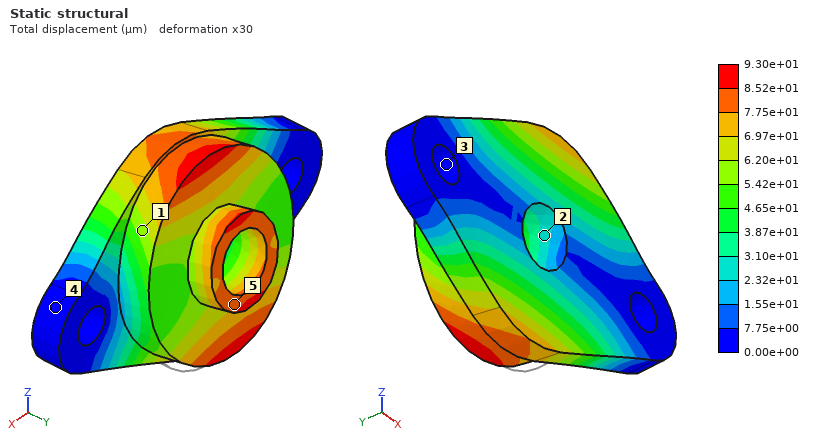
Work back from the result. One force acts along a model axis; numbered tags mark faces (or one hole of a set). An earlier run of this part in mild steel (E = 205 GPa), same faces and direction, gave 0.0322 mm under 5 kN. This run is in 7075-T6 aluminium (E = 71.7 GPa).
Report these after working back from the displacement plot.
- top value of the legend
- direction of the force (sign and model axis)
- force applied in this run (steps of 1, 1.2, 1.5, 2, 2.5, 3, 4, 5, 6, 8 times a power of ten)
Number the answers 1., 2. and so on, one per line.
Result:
1. 9.30e+01 µm
2. +Z
3. 5 kN
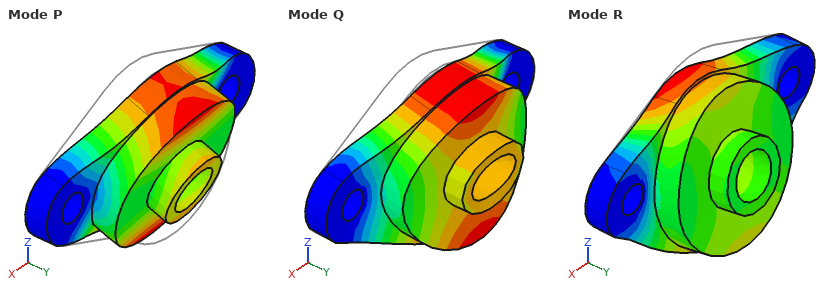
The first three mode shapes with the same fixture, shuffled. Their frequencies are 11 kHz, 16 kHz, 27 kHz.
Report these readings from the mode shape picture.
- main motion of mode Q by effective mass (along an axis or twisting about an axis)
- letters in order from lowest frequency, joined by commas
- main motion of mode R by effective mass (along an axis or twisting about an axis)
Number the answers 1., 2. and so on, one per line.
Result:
1. along Y
2. P, Q, R
3. along Z
